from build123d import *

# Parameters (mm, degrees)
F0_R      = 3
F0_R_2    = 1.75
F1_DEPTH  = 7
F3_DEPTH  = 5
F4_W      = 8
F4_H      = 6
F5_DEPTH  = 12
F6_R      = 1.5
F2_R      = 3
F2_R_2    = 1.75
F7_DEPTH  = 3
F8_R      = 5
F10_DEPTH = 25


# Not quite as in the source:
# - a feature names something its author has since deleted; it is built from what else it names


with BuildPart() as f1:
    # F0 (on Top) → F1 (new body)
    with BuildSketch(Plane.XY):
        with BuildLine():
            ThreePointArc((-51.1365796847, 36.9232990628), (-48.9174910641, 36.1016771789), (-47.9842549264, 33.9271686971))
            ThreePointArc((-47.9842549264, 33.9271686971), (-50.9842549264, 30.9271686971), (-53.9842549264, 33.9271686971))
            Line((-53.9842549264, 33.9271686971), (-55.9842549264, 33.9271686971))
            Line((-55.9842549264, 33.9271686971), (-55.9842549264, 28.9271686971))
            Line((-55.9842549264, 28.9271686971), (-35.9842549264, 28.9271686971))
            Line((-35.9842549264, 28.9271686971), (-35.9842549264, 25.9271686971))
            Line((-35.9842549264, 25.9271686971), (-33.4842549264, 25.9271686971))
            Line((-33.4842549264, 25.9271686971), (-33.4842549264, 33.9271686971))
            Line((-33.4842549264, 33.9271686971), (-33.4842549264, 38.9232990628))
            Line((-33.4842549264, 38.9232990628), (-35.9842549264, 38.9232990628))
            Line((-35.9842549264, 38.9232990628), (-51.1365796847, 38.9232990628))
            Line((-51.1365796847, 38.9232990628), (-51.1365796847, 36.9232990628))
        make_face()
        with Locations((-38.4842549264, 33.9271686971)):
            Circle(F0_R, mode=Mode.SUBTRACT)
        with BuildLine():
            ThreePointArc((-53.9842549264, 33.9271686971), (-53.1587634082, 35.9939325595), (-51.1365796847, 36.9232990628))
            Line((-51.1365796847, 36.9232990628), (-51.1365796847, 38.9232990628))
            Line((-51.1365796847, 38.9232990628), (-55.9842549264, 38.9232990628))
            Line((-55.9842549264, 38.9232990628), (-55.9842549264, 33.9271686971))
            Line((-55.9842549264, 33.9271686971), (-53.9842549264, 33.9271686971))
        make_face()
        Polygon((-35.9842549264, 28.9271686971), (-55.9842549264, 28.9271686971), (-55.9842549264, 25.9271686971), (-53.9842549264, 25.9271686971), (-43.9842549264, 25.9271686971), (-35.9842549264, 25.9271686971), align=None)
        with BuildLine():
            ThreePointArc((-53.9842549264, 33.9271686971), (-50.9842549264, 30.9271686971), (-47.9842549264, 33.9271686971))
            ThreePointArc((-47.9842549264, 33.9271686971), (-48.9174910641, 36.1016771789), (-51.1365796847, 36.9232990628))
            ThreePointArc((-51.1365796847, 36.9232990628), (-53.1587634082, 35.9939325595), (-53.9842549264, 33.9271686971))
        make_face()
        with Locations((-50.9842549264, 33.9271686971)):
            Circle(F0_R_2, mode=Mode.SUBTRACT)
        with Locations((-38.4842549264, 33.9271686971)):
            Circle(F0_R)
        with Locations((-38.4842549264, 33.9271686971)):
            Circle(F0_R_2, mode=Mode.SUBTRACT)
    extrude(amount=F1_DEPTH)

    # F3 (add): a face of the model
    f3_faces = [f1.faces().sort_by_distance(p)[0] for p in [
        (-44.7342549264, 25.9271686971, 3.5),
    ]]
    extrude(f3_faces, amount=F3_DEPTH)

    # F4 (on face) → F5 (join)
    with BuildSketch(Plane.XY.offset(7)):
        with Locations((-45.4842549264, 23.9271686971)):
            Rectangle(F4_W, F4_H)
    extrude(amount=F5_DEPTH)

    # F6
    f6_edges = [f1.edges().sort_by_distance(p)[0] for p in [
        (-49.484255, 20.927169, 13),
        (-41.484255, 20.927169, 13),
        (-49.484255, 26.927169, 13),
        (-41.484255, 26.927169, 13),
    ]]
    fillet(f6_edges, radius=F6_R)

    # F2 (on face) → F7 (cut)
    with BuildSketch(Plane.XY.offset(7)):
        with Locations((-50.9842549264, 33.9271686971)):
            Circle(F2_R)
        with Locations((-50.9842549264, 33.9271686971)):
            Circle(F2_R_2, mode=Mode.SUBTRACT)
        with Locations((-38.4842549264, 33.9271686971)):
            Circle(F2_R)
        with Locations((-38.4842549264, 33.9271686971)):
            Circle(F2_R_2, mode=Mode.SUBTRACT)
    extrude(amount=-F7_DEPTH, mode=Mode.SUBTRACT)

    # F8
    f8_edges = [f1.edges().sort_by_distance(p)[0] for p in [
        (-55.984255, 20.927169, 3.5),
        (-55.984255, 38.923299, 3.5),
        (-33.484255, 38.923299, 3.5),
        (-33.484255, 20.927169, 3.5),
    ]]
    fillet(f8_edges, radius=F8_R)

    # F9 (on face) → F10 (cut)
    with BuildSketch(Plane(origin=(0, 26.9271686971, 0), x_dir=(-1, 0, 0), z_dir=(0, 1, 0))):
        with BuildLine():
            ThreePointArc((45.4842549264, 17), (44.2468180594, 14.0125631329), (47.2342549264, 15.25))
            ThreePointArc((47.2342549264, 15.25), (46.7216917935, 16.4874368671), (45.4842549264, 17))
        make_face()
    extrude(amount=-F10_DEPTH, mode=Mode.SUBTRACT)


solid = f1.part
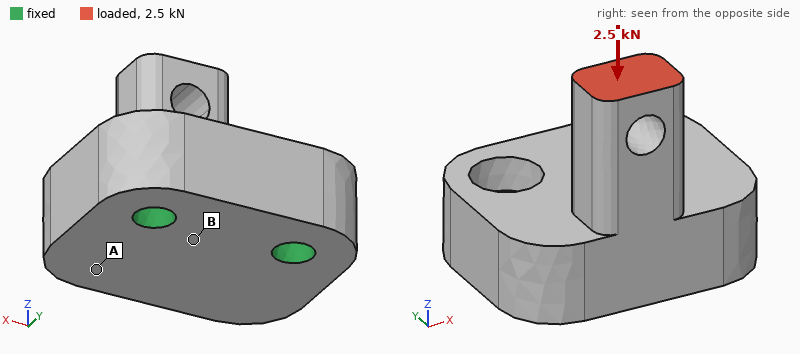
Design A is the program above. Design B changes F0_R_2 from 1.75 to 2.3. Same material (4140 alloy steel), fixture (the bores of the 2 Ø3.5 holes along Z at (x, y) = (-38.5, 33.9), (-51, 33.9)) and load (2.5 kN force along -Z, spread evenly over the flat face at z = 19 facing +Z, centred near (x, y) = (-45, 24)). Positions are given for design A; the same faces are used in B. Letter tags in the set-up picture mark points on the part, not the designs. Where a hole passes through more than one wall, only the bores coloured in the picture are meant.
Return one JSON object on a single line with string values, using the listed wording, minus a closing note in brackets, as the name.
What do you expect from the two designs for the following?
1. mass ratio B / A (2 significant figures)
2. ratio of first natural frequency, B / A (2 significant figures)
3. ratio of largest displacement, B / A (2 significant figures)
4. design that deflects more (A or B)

{"mass ratio B / A": "0.98", "ratio of first natural frequency, B / A": "1.1", "ratio of largest displacement, B / A": "0.80", "design that deflects more": "A"}
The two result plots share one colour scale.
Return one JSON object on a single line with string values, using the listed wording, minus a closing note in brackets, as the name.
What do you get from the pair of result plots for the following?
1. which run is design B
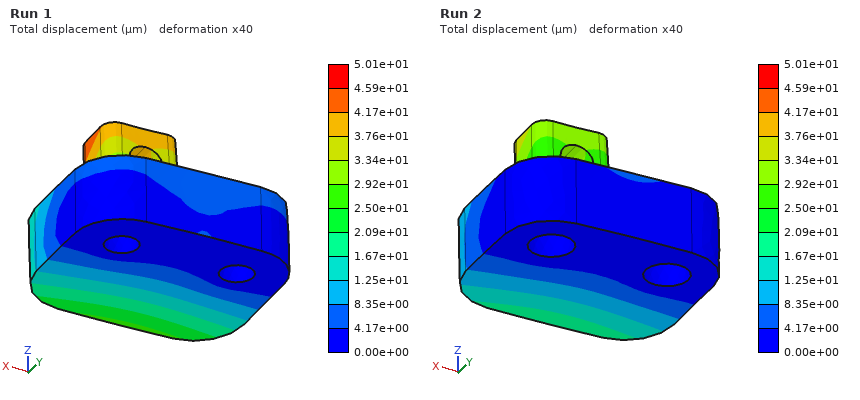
{"which run is design B": "Run 2"}
